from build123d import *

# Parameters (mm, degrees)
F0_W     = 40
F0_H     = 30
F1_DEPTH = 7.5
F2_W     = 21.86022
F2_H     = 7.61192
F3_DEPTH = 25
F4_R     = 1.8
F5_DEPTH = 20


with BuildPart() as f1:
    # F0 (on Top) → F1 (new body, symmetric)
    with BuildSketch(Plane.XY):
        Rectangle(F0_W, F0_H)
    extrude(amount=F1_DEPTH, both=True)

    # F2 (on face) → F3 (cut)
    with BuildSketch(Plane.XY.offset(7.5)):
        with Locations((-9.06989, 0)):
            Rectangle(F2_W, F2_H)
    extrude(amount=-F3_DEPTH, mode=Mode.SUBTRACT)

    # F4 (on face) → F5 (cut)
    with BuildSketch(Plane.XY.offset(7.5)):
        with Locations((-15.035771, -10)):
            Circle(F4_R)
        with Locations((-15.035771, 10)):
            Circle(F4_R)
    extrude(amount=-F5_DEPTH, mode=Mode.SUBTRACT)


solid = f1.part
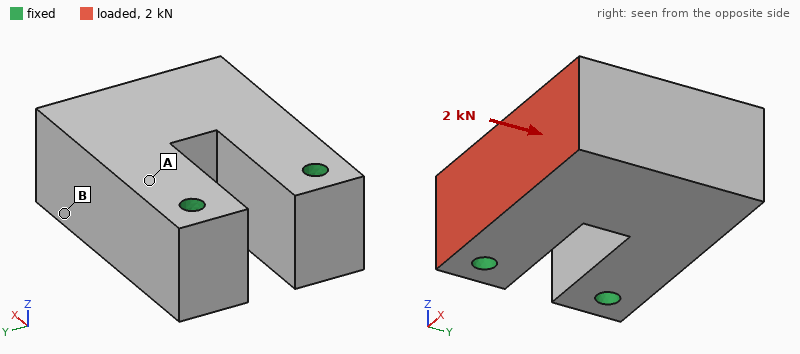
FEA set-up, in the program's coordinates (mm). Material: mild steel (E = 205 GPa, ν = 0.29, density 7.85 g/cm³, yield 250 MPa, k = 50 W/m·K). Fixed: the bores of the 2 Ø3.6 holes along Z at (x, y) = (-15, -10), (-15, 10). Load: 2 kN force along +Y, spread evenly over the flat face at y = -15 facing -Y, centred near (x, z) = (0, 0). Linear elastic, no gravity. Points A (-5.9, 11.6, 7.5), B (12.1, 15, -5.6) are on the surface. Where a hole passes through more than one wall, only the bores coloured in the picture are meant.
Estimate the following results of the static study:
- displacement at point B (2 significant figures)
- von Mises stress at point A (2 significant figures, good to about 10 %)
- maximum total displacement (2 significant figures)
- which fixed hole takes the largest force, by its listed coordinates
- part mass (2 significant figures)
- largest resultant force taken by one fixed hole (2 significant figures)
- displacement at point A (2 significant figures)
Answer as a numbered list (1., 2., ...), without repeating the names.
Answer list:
1. 4.2 µm
2. 11 MPa
3. 5.0 µm
4. (-15, -10)
5. 120 g
6. 1.7 kN
7. 1.7 µm
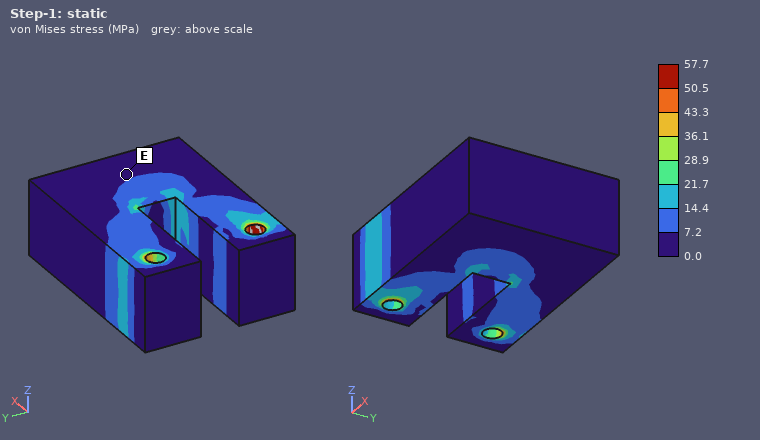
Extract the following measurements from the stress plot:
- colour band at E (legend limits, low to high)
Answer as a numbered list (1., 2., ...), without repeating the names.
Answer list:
1. 0.0 to 7.2 MPa
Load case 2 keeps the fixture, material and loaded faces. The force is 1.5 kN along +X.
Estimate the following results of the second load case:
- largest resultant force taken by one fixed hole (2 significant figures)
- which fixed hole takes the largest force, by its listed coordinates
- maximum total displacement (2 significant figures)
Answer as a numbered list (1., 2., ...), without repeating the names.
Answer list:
1. 1.7 kN
2. (-15, -10)
3. 2.4 µm
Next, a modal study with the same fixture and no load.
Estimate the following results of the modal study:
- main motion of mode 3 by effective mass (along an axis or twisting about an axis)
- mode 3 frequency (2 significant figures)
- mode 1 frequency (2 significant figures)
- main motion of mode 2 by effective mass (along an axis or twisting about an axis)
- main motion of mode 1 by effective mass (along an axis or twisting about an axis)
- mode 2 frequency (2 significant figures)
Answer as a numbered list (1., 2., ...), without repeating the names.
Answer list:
1. twisting about X
2. 16 kHz
3. 7700 Hz
4. along Y
5. along Z
6. 10 kHz
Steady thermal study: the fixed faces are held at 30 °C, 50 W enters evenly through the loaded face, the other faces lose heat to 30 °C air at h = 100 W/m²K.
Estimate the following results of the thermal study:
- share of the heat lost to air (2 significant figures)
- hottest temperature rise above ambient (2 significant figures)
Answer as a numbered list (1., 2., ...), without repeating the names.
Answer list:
1. 15 %
2. 49 K
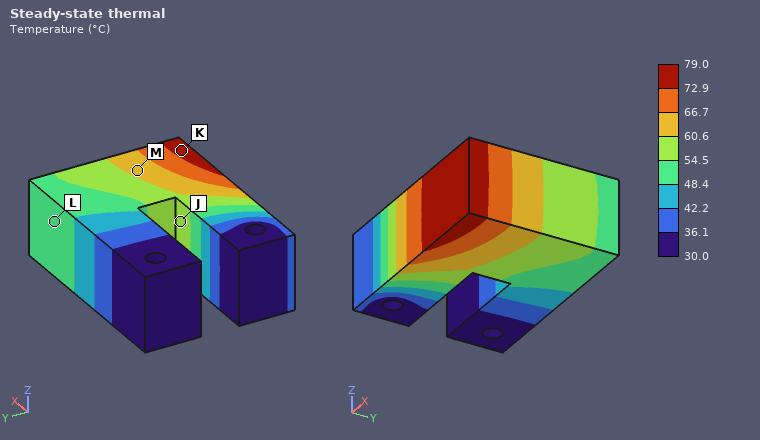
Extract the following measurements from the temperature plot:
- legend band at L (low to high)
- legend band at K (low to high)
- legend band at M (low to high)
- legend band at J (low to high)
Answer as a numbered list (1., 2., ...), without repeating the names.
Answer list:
1. 48.4 to 54.5 °C
2. 72.9 to 79.0 °C
3. 60.6 to 66.7 °C
4. 54.5 to 60.6 °C
